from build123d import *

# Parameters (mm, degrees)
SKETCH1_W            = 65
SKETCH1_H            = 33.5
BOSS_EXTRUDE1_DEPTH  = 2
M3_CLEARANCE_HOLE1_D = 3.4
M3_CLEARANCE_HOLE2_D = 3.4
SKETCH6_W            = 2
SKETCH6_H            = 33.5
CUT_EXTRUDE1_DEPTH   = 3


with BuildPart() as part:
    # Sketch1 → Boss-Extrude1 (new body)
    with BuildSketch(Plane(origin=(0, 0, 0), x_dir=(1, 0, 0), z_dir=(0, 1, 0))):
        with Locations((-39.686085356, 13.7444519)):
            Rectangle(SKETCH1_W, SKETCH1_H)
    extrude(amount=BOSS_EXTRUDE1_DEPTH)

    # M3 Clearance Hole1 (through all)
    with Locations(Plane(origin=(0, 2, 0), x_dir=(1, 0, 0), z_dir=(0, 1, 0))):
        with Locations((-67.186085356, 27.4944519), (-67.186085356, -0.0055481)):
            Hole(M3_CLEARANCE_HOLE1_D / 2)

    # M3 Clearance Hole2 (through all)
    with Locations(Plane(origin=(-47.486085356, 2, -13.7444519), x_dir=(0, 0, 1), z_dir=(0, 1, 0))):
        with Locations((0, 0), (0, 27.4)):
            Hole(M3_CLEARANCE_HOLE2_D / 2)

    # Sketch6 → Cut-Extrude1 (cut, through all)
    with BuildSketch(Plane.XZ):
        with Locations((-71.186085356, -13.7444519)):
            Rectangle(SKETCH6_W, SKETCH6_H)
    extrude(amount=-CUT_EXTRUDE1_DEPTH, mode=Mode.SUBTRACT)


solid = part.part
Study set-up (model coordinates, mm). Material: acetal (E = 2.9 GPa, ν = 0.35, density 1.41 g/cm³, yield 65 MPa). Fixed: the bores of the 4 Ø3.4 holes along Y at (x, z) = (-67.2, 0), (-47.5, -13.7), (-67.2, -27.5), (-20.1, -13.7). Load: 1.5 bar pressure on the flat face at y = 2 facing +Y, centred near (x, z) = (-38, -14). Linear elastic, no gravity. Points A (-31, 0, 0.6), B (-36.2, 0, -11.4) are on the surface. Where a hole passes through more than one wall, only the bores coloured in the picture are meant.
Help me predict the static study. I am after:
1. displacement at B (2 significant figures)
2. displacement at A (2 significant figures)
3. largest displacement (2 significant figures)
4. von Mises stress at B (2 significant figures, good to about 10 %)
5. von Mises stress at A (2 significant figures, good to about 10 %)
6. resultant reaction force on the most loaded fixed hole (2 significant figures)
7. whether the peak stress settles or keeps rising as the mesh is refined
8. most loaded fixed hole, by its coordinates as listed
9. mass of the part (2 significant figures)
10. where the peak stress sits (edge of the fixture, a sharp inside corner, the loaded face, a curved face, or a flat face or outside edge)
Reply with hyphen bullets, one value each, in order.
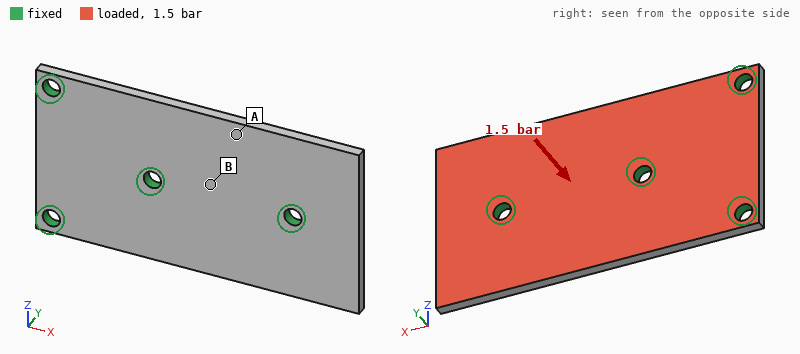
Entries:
- 0.16 mm
- 0.54 mm
- 0.72 mm
- 14 MPa
- 4.4 MPa
- 140 N
- keeps rising
- (-20.1, -13.7)
- 5.8 g
- edge of the fixture
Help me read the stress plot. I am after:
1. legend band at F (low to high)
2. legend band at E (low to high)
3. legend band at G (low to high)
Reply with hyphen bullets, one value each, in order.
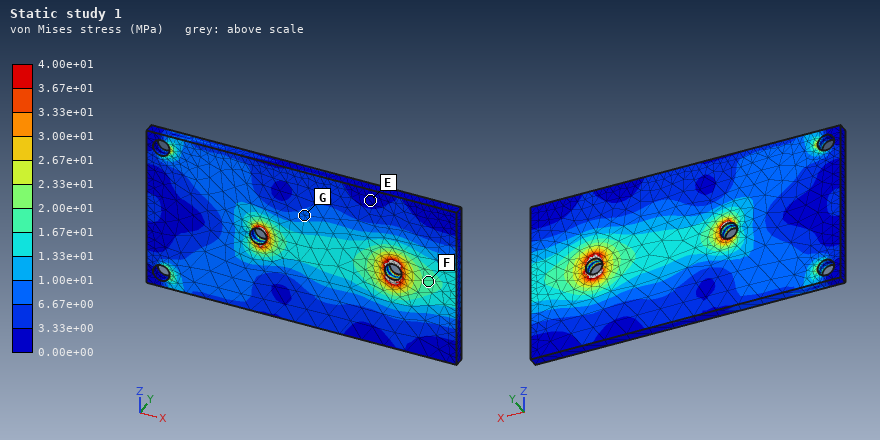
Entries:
- 1.67e+01 to 2.00e+01 MPa
- 0.00e+00 to 3.33e+00 MPa
- 6.67e+00 to 1.00e+01 MPa
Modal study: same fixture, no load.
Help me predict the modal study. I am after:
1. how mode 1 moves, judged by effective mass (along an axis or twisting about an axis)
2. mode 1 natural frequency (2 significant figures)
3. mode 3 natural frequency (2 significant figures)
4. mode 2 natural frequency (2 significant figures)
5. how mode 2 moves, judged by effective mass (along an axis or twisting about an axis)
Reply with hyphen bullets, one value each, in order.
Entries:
- twisting about X
- 1400 Hz
- 2000 Hz
- 1800 Hz
- along Y
